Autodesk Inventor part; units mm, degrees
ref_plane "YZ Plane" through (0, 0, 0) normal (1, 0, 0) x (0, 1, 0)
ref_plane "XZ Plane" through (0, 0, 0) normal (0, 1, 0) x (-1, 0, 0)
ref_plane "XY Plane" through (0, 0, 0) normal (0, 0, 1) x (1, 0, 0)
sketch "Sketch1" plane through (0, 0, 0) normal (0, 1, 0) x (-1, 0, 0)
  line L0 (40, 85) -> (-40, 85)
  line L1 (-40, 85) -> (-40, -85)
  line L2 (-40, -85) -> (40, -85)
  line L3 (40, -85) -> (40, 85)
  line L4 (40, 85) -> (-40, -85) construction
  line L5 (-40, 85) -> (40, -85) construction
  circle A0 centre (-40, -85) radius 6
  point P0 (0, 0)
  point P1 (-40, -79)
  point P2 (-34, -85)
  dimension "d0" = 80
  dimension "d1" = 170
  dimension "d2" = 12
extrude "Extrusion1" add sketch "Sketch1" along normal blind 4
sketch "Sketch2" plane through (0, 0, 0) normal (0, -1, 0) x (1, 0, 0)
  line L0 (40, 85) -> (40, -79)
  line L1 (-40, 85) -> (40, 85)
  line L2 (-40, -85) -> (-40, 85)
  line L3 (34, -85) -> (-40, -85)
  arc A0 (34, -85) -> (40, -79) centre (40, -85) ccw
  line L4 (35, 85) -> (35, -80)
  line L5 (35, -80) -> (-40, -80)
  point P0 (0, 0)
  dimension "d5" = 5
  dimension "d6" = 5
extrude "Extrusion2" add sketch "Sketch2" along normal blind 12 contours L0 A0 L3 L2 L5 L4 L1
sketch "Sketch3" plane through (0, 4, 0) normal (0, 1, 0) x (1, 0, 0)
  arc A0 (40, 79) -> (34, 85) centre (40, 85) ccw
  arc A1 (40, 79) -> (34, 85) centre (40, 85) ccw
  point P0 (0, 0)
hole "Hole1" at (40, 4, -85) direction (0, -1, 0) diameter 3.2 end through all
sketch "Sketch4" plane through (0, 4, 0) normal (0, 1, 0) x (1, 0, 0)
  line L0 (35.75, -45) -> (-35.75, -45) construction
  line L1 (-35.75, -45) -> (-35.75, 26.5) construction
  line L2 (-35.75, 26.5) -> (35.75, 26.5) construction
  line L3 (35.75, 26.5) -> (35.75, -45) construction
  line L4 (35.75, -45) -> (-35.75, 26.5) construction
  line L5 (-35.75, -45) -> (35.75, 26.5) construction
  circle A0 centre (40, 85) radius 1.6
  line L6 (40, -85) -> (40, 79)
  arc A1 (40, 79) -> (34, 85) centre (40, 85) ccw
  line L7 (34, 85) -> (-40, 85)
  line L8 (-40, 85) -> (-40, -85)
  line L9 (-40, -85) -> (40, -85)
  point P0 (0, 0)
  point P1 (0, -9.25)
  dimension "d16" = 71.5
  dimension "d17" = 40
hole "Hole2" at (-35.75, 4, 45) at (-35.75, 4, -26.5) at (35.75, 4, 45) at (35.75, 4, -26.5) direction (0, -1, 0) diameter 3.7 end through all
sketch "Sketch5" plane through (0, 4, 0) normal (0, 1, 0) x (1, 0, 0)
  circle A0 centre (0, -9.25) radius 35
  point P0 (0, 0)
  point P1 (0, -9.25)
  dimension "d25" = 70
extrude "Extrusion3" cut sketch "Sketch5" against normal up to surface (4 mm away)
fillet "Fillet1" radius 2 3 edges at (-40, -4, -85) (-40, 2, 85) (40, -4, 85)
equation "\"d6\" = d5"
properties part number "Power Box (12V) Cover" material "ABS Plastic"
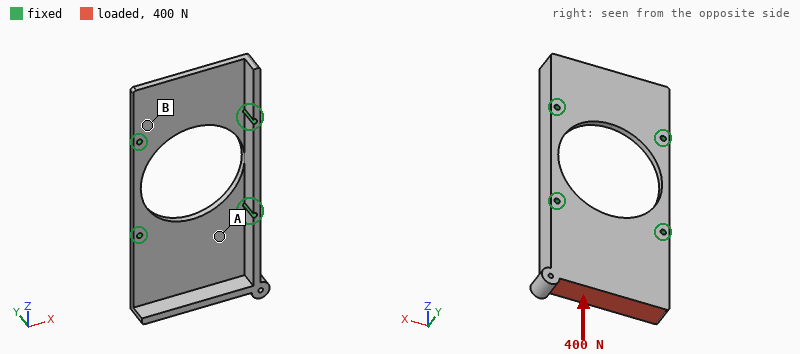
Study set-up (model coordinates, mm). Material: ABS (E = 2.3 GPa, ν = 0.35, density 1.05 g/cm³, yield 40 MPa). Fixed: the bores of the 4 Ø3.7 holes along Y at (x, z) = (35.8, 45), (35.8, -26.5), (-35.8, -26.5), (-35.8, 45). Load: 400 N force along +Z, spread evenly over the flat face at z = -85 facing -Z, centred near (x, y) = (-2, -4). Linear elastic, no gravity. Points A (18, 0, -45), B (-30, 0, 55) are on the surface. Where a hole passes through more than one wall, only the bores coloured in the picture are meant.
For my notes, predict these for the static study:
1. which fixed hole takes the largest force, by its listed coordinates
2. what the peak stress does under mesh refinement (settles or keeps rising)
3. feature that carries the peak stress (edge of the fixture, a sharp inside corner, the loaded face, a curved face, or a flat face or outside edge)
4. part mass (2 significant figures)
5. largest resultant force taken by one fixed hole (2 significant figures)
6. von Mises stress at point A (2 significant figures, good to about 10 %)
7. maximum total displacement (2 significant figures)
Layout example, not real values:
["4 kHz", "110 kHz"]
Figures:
["(-35.8, -26.5)", "keeps rising", "edge of the fixture", "57 g", "220 N", "3.0 MPa", "2.2 mm"]
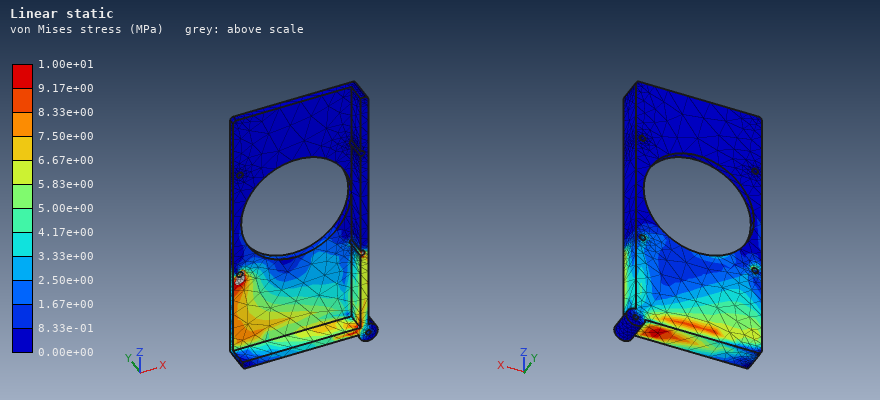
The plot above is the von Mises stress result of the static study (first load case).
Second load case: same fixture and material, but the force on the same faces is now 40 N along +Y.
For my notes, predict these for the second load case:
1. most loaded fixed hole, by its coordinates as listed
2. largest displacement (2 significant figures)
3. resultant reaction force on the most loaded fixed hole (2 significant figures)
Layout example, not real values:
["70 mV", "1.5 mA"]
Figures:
["(35.8, -26.5)", "1.9 mm", "25 N"]
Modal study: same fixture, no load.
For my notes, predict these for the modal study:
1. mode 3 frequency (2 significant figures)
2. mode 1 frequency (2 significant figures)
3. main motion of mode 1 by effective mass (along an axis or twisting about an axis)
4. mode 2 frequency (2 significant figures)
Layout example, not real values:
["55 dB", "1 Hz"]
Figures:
["700 Hz", "270 Hz", "along Y", "550 Hz"]
